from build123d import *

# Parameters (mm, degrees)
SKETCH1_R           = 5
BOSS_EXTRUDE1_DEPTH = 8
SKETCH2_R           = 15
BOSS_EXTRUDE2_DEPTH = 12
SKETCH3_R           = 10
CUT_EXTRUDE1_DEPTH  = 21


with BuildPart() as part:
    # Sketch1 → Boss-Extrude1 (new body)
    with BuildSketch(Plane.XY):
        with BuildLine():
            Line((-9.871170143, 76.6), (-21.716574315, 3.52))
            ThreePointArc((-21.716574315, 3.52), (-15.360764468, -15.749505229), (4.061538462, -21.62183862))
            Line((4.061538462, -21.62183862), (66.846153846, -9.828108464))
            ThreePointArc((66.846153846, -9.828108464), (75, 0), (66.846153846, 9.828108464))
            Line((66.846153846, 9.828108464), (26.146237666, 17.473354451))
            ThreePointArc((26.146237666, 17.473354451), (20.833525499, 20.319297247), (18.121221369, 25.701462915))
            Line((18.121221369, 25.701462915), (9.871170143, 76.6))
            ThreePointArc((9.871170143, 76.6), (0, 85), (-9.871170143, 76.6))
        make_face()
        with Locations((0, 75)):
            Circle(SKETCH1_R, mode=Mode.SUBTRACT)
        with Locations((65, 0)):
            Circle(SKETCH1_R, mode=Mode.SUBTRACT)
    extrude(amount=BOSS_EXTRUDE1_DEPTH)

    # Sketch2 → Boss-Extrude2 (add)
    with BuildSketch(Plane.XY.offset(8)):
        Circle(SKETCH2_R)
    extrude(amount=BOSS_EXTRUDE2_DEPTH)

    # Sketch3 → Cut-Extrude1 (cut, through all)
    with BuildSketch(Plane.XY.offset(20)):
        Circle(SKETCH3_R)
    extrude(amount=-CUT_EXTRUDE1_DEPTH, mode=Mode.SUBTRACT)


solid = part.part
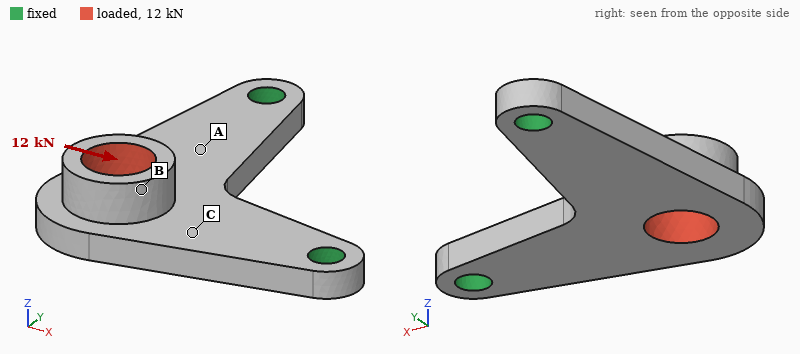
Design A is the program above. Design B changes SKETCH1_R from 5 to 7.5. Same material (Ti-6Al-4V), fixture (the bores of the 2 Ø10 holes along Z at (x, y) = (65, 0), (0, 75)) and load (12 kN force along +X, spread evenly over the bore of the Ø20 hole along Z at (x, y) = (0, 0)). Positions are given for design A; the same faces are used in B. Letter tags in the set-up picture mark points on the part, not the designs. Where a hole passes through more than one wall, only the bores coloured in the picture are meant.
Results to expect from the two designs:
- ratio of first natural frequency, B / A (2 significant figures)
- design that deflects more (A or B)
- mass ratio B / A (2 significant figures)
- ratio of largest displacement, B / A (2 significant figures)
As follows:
1.1
A
0.96
0.90
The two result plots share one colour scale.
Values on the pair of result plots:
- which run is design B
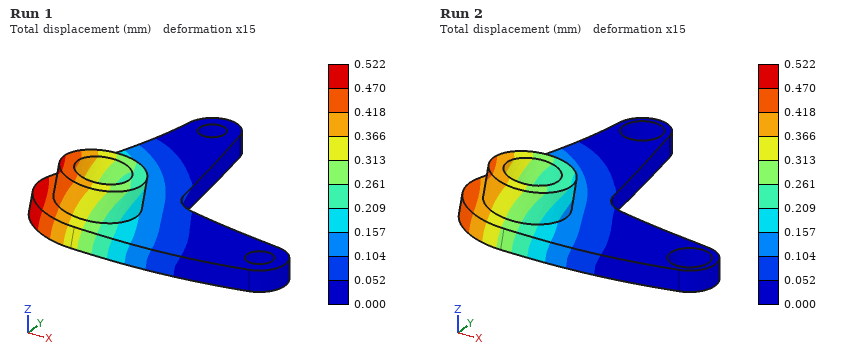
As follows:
Run 2
